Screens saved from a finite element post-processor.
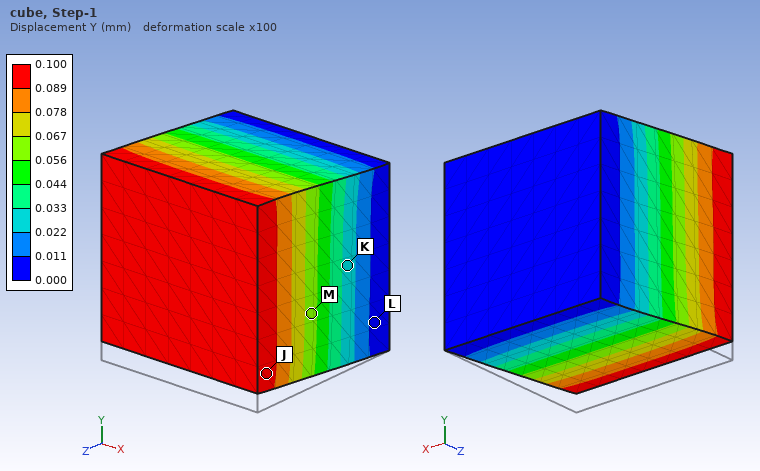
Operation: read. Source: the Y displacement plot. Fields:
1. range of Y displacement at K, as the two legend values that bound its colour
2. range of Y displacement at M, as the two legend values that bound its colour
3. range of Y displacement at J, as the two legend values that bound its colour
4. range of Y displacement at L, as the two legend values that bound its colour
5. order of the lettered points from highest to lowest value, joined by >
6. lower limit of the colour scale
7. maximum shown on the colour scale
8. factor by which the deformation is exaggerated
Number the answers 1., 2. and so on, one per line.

1. 0.022 to 0.033 mm
2. 0.056 to 0.067 mm
3. 0.089 to 0.100 mm
4. 0.000 to 0.011 mm
5. J > M > K > L
6. 0.000 mm
7. 0.100 mm
8. 100
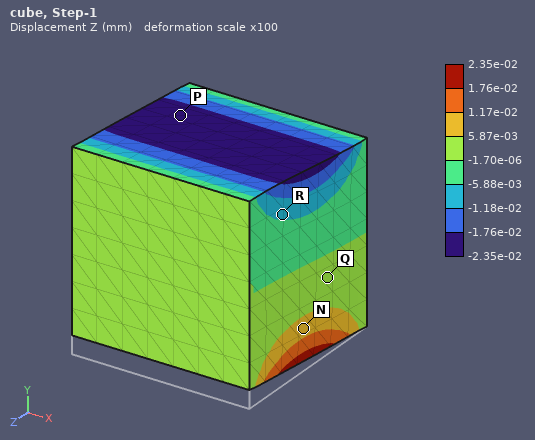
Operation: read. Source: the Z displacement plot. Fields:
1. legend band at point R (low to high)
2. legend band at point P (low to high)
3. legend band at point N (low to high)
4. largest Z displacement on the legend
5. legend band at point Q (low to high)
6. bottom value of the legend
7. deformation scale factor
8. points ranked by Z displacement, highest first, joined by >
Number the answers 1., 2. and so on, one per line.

1. -1.18e-02 to -5.88e-03 mm
2. -2.35e-02 to -1.76e-02 mm
3. 5.87e-03 to 1.17e-02 mm
4. 2.35e-02 mm
5. -1.70e-06 to 5.87e-03 mm
6. -2.35e-02 mm
7. 100
8. N > Q > R > P
